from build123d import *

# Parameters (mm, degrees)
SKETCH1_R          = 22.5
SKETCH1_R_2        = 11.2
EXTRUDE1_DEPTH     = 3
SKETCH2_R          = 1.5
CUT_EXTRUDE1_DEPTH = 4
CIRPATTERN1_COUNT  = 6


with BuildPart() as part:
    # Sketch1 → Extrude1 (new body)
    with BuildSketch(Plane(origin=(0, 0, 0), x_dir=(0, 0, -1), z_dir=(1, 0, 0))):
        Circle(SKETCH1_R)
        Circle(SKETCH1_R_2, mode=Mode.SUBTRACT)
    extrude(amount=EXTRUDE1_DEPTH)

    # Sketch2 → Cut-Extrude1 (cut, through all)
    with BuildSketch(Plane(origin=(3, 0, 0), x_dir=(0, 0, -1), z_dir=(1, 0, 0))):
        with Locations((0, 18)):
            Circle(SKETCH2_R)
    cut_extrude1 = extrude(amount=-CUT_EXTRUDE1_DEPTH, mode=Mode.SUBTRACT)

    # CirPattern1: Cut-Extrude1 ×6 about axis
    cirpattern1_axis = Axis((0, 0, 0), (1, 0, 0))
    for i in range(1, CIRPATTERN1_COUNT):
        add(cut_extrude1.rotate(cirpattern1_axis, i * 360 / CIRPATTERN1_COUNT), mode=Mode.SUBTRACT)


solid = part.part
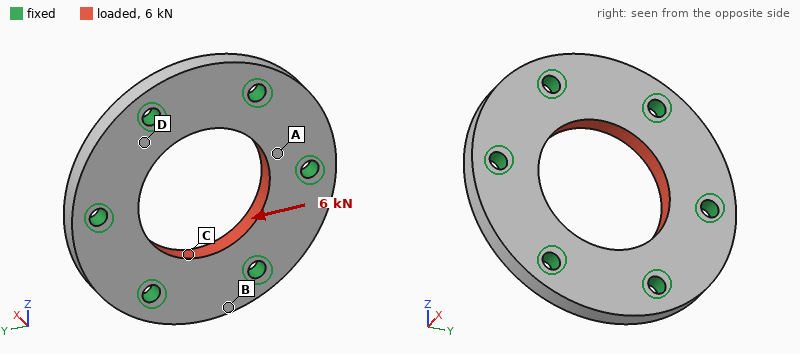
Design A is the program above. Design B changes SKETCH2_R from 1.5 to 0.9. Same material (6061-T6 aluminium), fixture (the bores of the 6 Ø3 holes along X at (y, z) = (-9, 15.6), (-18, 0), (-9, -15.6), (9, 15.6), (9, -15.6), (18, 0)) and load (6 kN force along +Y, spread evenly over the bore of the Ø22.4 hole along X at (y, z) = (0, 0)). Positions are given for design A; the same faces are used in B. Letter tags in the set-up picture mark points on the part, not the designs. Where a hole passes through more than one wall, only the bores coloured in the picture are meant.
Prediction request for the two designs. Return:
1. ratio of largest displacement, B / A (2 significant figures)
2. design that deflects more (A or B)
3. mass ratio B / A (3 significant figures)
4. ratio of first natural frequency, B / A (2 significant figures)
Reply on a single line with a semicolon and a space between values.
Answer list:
1.2; B; 1.02; 0.83
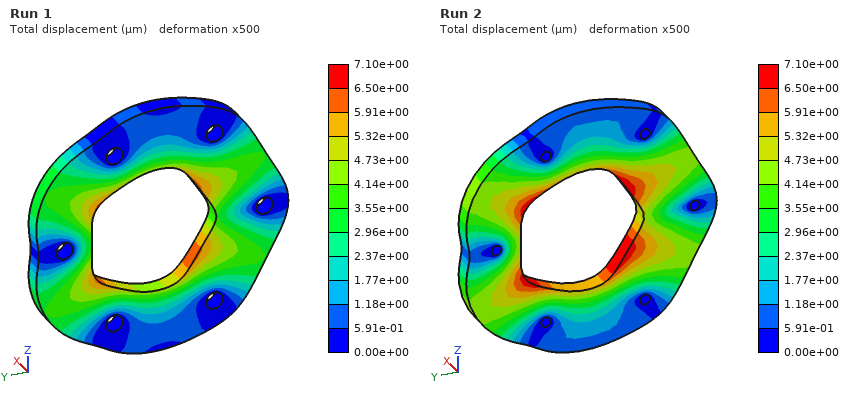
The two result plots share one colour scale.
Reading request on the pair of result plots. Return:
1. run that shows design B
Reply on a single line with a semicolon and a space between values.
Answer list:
Run 2
